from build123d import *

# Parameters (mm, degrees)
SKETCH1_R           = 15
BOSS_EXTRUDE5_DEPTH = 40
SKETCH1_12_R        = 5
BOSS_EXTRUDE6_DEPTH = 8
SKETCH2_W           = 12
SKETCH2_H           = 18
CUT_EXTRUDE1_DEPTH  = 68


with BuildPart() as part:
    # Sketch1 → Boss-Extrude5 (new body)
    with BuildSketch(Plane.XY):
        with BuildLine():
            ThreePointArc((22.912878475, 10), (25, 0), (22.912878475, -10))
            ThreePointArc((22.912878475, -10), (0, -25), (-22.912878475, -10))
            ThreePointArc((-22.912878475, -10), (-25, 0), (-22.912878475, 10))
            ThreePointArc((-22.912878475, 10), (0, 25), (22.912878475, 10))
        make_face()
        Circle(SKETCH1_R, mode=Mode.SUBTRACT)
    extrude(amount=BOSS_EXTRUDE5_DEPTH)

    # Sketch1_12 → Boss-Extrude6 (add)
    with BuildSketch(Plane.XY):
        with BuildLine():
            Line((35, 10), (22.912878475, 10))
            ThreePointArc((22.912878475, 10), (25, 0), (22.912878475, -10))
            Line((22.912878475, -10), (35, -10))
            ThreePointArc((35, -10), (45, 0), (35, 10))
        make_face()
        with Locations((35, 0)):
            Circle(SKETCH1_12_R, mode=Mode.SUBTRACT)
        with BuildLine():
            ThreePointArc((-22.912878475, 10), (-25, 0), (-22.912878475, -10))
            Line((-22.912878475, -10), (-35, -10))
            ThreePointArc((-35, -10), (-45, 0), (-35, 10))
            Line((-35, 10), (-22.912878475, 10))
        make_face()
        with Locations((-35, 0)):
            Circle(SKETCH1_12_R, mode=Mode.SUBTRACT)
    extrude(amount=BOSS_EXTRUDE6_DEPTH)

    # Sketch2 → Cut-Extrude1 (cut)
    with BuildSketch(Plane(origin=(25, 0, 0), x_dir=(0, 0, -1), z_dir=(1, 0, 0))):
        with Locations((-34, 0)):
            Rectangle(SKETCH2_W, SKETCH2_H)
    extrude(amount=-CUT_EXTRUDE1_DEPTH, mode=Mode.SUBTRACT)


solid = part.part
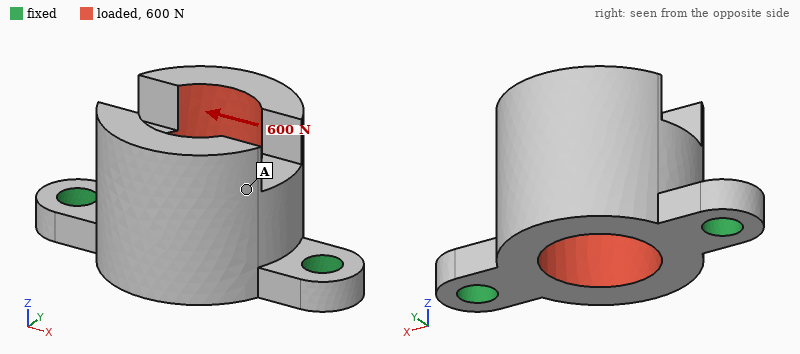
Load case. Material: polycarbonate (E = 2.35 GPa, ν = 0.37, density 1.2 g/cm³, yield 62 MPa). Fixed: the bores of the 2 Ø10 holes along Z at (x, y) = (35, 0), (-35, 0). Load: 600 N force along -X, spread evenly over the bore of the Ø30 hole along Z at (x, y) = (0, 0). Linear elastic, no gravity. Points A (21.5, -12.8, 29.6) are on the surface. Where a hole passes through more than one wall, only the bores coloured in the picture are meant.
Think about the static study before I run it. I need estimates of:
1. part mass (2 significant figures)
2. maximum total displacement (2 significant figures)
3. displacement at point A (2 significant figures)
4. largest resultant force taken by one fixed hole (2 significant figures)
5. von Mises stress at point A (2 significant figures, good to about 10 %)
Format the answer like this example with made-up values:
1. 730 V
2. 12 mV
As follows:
1. 61 g
2. 58 µm
3. 45 µm
4. 340 N
5. 0.70 MPa
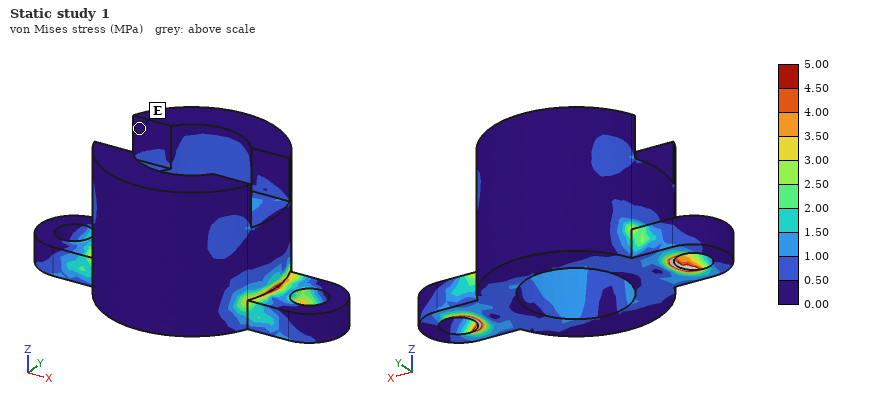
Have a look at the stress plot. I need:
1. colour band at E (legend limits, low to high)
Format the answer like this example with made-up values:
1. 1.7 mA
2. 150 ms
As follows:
1. 0.00 to 0.50 MPa
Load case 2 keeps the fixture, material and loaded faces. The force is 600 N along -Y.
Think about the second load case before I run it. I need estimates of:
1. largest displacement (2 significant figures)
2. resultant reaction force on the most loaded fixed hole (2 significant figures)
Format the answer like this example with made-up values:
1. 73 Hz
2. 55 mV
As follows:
1. 0.71 mm
2. 300 N
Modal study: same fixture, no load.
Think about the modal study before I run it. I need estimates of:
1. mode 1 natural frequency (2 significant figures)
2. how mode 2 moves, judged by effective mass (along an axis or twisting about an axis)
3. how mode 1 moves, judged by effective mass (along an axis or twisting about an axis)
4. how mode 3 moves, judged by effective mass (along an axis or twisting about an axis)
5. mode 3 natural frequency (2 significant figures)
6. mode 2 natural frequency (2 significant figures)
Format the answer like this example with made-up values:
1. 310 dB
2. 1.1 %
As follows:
1. 660 Hz
2. along Z
3. along Y
4. along X
5. 2600 Hz
6. 2000 Hz
